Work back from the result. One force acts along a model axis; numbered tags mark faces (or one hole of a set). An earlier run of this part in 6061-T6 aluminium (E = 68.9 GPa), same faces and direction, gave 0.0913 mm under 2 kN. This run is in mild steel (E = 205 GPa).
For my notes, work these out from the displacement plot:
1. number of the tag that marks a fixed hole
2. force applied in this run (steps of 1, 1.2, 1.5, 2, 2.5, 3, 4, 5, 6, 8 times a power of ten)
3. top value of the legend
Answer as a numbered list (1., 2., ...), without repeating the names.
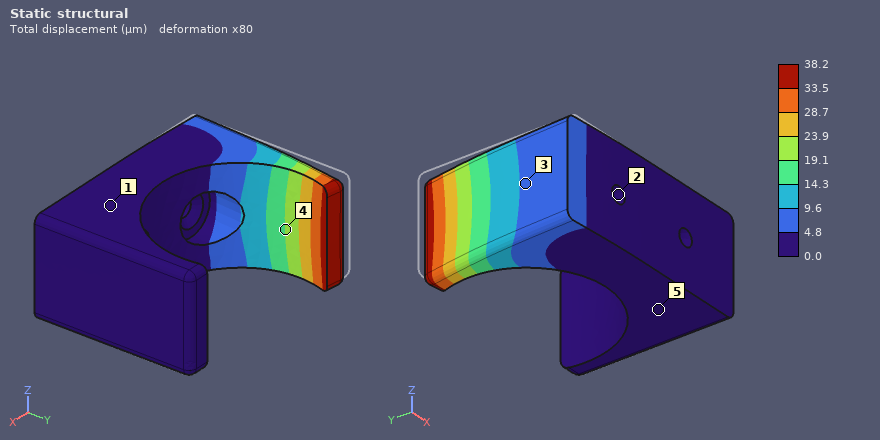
1. 2
2. 2.5 kN
3. 38.2 µm
